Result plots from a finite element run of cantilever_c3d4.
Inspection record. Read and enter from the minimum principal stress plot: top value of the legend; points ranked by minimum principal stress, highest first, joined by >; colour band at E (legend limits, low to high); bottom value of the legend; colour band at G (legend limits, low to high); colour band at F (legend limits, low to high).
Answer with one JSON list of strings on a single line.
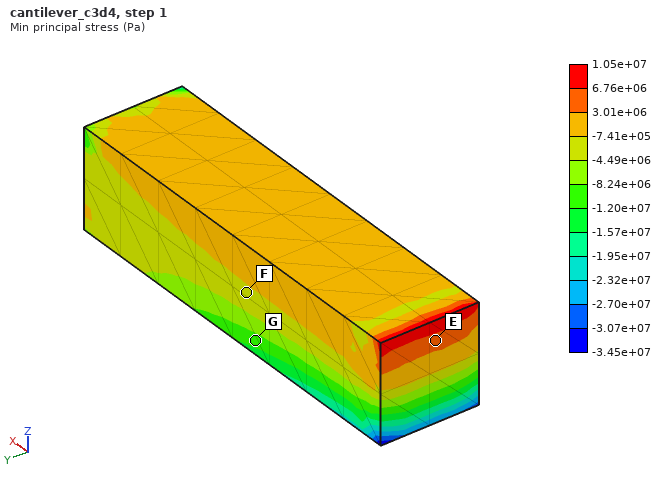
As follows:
["1.05e+07 Pa", "E > F > G", "3.01e+06 to 6.76e+06 Pa", "-3.45e+07 Pa", "-1.20e+07 to -8.24e+06 Pa", "-4.49e+06 to -7.41e+05 Pa"]
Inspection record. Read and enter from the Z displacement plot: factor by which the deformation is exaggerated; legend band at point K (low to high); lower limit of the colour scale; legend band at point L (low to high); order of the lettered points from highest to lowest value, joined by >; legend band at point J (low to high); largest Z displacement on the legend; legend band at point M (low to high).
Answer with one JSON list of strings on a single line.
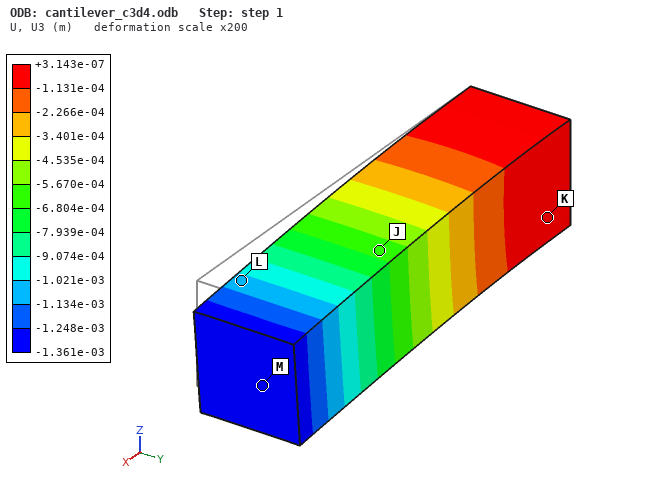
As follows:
["200", "-1.131e-04 to +3.143e-07 m", "-1.361e-03 m", "-1.134e-03 to -1.021e-03 m", "K > J > L > M", "-6.804e-04 to -5.670e-04 m", "+3.143e-07 m", "-1.361e-03 to -1.248e-03 m"]
